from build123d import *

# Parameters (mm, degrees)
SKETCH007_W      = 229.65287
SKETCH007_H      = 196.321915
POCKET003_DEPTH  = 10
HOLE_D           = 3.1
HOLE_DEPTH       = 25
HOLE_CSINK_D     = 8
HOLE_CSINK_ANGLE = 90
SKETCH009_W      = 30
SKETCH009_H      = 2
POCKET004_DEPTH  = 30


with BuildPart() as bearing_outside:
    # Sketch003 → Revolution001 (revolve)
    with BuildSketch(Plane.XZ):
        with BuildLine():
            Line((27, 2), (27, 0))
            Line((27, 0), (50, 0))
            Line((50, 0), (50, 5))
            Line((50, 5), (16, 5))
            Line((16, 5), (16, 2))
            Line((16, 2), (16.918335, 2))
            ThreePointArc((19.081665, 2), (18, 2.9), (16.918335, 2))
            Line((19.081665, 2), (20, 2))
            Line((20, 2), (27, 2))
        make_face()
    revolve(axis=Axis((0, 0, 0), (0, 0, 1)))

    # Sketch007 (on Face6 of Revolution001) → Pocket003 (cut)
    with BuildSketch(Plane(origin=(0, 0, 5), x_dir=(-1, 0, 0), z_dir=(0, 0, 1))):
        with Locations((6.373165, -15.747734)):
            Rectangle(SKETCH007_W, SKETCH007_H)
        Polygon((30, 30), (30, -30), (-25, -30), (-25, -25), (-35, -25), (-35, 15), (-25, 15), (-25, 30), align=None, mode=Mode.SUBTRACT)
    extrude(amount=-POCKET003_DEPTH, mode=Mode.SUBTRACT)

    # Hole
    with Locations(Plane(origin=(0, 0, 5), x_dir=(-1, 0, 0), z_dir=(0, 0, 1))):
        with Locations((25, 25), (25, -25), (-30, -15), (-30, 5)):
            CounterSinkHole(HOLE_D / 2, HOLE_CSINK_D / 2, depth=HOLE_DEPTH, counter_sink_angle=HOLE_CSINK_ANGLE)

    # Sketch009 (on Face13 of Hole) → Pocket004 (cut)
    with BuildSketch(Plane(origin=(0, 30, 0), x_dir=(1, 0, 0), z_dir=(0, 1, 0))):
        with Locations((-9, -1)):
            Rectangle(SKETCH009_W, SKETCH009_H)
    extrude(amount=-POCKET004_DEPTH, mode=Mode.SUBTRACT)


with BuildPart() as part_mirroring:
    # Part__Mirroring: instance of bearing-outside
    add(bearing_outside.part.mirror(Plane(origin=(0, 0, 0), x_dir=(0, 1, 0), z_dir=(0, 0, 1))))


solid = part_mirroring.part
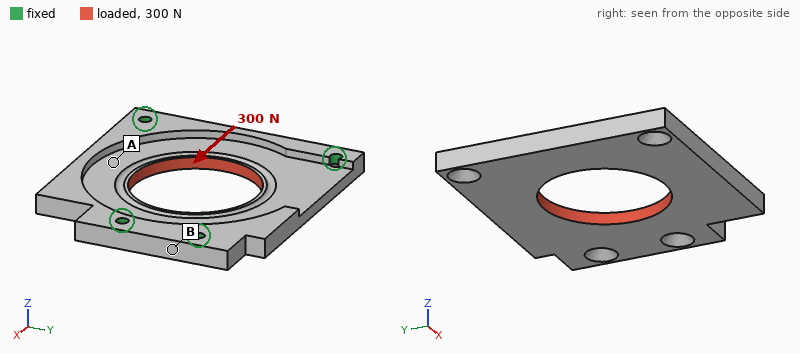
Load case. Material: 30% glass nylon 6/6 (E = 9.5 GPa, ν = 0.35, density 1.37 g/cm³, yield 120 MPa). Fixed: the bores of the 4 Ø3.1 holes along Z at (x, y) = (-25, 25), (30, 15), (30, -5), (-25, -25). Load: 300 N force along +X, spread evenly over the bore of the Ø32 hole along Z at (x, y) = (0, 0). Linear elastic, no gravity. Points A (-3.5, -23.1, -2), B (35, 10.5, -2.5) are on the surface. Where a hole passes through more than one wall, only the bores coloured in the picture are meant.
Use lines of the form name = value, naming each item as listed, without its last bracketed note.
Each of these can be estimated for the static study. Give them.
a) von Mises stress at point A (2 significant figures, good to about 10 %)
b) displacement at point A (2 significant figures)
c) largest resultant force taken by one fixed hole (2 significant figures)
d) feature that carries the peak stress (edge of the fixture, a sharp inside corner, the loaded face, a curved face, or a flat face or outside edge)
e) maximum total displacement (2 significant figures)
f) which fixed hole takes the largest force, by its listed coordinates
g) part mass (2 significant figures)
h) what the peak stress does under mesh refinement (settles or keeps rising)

von Mises stress at point A = 2.0 MPa
displacement at point A = 11 µm
largest resultant force taken by one fixed hole = 100 N
feature that carries the peak stress = edge of the fixture
maximum total displacement = 19 µm
which fixed hole takes the largest force, by its listed coordinates = (-25, -25)
part mass = 15 g
what the peak stress does under mesh refinement = keeps rising
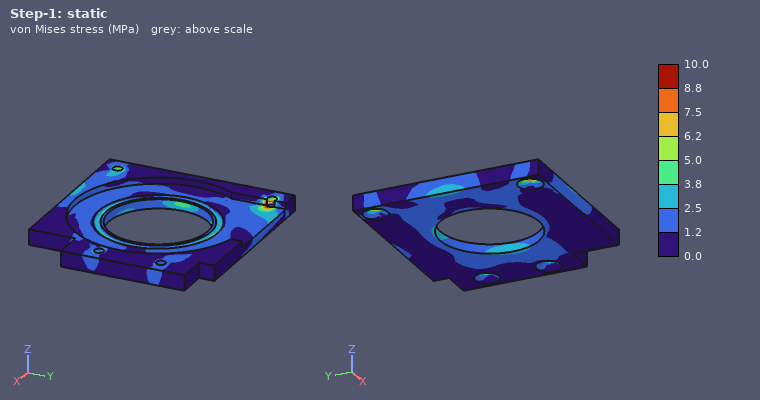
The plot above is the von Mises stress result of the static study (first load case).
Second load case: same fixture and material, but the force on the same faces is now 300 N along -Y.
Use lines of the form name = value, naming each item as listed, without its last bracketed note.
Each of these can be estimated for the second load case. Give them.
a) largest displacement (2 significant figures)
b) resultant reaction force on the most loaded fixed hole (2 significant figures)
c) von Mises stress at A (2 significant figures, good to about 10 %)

largest displacement = 16 µm
resultant reaction force on the most loaded fixed hole = 83 N
von Mises stress at A = 0.90 MPa
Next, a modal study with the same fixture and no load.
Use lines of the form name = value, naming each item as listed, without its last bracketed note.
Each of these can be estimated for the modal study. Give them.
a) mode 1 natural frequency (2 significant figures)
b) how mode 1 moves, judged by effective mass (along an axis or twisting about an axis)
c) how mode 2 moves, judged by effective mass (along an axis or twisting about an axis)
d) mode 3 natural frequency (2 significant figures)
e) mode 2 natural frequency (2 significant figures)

mode 1 natural frequency = 2300 Hz
how mode 1 moves, judged by effective mass = along Z
how mode 2 moves, judged by effective mass = along Z
mode 3 natural frequency = 3800 Hz
mode 2 natural frequency = 2700 Hz
